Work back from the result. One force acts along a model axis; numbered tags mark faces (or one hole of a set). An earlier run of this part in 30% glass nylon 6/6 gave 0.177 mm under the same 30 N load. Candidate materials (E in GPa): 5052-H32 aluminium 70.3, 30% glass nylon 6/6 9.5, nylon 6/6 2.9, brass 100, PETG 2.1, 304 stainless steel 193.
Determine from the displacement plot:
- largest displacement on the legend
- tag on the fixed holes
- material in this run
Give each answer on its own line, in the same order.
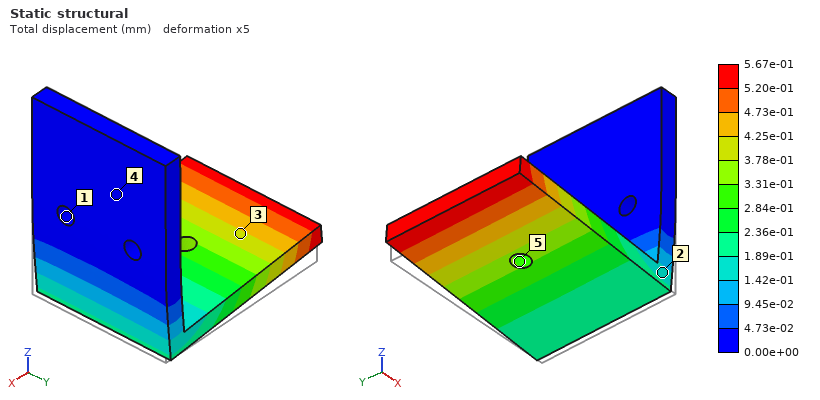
5.67e-01 mm
1
nylon 6/6
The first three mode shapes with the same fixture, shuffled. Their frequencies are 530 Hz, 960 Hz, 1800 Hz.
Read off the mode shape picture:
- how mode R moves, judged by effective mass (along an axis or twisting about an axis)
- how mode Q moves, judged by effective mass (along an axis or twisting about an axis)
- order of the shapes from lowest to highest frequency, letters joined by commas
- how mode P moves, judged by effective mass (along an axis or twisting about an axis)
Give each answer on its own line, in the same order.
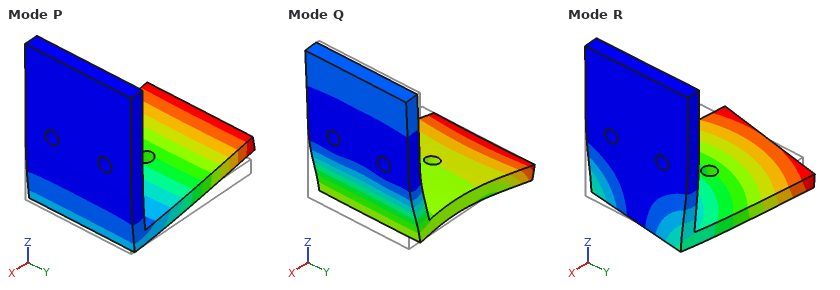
along Y
along X
P, R, Q
along Z
